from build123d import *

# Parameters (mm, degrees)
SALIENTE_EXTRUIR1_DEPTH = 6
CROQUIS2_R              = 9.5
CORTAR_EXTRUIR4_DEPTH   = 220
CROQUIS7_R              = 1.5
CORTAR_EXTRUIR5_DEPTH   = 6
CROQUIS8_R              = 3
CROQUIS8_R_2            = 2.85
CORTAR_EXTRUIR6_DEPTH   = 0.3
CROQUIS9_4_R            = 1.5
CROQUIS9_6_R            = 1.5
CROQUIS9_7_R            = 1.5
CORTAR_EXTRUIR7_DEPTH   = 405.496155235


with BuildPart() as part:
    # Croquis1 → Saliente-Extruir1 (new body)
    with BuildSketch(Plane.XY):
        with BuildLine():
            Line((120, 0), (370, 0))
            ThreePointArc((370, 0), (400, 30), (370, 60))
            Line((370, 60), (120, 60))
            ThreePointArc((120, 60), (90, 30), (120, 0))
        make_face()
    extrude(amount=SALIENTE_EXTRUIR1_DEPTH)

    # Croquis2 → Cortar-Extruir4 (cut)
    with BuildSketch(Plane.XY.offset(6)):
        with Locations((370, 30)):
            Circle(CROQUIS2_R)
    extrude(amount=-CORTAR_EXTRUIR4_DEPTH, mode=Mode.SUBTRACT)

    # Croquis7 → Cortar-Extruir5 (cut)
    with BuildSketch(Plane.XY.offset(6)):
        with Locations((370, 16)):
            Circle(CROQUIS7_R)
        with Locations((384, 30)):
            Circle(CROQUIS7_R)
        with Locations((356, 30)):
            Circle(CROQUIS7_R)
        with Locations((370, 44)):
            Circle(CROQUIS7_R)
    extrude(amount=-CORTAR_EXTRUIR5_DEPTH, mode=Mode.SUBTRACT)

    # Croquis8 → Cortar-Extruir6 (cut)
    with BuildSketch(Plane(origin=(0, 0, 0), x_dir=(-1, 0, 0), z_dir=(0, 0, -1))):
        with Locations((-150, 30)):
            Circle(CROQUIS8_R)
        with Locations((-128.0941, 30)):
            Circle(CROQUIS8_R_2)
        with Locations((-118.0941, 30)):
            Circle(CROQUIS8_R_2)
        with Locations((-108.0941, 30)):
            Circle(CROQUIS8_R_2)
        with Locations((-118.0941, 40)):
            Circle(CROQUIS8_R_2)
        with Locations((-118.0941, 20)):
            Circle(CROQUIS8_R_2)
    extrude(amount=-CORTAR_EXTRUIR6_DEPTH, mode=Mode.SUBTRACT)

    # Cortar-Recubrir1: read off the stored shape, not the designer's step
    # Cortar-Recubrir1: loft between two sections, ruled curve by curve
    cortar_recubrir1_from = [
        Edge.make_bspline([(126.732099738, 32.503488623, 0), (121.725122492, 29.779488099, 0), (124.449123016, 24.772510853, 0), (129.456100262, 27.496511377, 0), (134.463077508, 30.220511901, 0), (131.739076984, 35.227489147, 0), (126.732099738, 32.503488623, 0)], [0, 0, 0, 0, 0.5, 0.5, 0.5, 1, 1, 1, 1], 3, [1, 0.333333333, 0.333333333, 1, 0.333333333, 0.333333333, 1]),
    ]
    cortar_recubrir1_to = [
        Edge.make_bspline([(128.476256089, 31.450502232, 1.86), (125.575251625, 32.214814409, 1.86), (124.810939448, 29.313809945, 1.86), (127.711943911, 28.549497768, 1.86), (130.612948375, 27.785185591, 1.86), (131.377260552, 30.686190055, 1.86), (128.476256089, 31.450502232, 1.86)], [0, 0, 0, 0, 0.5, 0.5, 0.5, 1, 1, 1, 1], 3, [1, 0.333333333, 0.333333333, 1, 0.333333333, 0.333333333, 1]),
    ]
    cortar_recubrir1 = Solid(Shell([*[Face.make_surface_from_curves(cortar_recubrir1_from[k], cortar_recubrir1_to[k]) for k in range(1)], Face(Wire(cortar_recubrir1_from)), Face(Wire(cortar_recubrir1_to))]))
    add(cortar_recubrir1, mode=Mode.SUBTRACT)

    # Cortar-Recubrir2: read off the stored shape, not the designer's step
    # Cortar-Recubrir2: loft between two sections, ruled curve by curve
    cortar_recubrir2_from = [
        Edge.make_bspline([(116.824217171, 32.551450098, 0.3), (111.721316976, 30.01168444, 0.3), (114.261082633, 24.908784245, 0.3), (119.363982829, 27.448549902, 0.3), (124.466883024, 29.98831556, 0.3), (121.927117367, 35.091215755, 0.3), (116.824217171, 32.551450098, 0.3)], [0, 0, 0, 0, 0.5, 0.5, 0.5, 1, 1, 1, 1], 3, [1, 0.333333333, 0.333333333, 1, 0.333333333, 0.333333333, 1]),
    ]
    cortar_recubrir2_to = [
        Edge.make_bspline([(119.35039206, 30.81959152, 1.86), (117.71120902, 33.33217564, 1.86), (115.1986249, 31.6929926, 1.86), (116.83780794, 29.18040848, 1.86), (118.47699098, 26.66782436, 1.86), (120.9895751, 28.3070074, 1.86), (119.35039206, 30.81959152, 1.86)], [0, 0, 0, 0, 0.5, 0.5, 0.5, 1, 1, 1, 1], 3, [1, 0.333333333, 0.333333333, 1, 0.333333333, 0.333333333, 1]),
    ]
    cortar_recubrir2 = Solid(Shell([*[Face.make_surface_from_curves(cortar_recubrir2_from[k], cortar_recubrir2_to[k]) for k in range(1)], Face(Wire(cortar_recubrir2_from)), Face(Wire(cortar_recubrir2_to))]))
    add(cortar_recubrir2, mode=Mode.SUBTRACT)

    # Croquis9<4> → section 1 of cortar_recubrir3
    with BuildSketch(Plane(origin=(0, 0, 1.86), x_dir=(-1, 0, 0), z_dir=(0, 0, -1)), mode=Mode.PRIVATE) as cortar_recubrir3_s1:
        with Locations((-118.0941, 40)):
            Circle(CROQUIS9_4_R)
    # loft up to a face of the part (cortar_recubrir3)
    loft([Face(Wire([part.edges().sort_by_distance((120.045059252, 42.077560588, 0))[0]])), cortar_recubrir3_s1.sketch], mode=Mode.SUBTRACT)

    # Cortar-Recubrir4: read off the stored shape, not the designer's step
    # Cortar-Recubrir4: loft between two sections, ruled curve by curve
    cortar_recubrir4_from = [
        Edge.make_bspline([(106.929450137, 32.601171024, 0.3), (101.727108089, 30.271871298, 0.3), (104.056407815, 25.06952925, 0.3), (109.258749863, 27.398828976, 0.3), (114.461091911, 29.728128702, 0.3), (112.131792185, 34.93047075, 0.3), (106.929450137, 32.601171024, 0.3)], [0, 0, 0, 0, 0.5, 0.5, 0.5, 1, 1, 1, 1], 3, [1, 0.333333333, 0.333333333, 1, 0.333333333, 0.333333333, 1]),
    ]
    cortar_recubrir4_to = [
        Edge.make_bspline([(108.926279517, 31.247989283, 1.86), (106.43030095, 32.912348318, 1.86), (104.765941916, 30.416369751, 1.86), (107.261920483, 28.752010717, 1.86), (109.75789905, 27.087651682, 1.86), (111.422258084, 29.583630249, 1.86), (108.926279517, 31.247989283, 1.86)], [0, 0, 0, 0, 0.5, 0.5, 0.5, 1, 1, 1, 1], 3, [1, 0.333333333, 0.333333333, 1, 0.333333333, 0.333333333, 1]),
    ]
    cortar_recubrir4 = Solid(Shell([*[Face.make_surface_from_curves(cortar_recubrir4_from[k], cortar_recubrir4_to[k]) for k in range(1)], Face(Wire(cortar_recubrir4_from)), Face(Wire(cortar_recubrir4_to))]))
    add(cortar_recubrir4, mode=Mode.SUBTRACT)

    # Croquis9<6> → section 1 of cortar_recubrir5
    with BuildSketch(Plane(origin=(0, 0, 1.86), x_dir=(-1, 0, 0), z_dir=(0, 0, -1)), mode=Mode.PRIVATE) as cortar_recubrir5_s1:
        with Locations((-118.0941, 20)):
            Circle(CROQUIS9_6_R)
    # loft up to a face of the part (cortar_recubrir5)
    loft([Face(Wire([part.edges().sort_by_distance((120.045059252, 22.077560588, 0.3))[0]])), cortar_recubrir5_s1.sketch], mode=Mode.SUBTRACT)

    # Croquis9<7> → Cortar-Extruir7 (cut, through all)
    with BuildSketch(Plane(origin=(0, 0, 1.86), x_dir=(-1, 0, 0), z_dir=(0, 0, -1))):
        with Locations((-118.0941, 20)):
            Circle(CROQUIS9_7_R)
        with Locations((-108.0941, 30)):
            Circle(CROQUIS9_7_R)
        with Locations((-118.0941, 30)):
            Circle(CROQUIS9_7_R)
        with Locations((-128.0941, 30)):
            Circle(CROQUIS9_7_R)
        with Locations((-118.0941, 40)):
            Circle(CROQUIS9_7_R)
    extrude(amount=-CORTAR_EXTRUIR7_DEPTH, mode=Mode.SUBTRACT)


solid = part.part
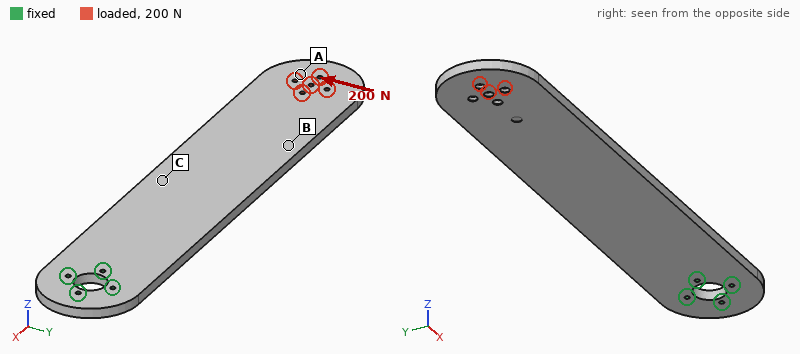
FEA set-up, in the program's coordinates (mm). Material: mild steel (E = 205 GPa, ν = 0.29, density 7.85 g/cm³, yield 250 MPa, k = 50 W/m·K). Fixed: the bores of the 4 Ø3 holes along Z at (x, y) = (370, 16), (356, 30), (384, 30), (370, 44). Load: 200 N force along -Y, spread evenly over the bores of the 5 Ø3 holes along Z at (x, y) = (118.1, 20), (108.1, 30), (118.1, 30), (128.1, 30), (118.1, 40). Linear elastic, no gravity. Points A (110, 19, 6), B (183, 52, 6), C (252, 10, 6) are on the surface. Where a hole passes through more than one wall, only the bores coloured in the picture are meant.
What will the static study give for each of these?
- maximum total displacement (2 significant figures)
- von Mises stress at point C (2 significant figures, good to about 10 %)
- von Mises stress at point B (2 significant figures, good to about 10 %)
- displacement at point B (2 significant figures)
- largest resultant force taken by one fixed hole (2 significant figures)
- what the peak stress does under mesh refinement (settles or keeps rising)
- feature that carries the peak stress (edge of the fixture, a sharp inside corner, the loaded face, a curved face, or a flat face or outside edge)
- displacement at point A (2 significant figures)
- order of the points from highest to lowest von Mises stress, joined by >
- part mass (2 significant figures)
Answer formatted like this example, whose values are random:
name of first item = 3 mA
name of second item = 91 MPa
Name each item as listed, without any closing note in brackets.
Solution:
maximum total displacement = 67 µm
von Mises stress at point C = 5.1 MPa
von Mises stress at point B = 2.9 MPa
displacement at point B = 38 µm
largest resultant force taken by one fixed hole = 1.1 kN
what the peak stress does under mesh refinement = keeps rising
feature that carries the peak stress = edge of the fixture
displacement at point A = 60 µm
order of the points from highest to lowest von Mises stress, joined by > = C > B > A
part mass = 820 g
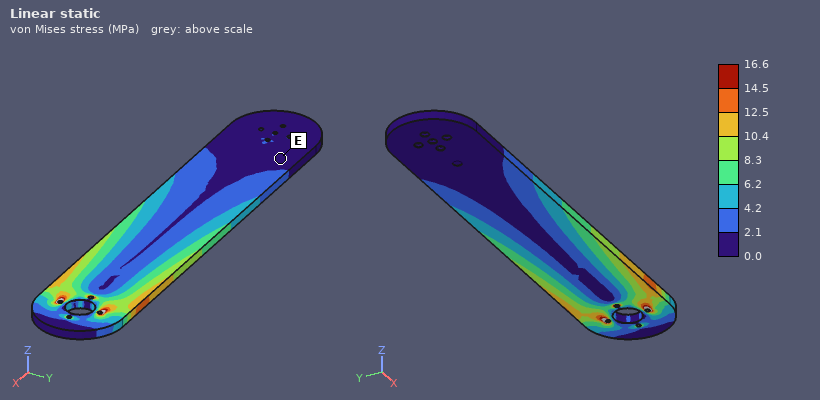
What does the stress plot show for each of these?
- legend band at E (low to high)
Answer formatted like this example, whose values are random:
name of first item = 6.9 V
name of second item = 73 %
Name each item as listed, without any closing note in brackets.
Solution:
legend band at E = 0.0 to 2.1 MPa
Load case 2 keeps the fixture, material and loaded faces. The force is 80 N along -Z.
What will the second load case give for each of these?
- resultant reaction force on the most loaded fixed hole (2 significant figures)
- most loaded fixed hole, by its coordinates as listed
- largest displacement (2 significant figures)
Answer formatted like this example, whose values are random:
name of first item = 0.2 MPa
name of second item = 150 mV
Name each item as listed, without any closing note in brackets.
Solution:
resultant reaction force on the most loaded fixed hole = 800 N
most loaded fixed hole, by its coordinates as listed = (356, 30)
largest displacement = 2.0 mm
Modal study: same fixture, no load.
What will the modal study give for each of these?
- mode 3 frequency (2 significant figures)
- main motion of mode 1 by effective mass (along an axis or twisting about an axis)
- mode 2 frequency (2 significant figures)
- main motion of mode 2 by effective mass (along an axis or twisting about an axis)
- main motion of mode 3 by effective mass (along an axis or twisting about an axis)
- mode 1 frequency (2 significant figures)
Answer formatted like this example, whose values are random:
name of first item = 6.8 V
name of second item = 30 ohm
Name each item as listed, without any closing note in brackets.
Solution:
mode 3 frequency = 590 Hz
main motion of mode 1 by effective mass = along Z
mode 2 frequency = 440 Hz
main motion of mode 2 by effective mass = along Z
main motion of mode 3 by effective mass = along Y
mode 1 frequency = 72 Hz
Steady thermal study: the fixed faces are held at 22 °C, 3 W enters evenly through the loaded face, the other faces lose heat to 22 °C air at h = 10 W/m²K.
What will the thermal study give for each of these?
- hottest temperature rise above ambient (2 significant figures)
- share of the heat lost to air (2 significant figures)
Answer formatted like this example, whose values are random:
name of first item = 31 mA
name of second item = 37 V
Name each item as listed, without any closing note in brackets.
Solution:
hottest temperature rise above ambient = 17 K
share of the heat lost to air = 80 %
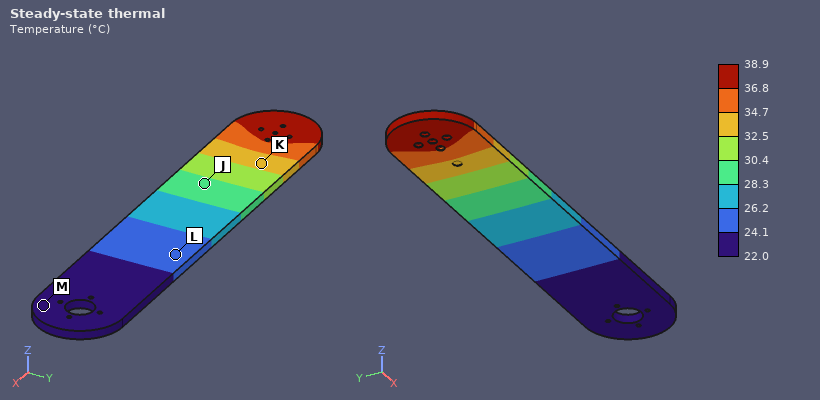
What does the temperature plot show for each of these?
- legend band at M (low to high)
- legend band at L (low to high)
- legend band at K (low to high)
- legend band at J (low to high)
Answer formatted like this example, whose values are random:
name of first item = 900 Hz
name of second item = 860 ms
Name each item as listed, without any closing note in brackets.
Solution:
legend band at M = 22.0 to 24.1 °C
legend band at L = 24.1 to 26.2 °C
legend band at K = 32.5 to 34.7 °C
legend band at J = 28.3 to 30.4 °C
